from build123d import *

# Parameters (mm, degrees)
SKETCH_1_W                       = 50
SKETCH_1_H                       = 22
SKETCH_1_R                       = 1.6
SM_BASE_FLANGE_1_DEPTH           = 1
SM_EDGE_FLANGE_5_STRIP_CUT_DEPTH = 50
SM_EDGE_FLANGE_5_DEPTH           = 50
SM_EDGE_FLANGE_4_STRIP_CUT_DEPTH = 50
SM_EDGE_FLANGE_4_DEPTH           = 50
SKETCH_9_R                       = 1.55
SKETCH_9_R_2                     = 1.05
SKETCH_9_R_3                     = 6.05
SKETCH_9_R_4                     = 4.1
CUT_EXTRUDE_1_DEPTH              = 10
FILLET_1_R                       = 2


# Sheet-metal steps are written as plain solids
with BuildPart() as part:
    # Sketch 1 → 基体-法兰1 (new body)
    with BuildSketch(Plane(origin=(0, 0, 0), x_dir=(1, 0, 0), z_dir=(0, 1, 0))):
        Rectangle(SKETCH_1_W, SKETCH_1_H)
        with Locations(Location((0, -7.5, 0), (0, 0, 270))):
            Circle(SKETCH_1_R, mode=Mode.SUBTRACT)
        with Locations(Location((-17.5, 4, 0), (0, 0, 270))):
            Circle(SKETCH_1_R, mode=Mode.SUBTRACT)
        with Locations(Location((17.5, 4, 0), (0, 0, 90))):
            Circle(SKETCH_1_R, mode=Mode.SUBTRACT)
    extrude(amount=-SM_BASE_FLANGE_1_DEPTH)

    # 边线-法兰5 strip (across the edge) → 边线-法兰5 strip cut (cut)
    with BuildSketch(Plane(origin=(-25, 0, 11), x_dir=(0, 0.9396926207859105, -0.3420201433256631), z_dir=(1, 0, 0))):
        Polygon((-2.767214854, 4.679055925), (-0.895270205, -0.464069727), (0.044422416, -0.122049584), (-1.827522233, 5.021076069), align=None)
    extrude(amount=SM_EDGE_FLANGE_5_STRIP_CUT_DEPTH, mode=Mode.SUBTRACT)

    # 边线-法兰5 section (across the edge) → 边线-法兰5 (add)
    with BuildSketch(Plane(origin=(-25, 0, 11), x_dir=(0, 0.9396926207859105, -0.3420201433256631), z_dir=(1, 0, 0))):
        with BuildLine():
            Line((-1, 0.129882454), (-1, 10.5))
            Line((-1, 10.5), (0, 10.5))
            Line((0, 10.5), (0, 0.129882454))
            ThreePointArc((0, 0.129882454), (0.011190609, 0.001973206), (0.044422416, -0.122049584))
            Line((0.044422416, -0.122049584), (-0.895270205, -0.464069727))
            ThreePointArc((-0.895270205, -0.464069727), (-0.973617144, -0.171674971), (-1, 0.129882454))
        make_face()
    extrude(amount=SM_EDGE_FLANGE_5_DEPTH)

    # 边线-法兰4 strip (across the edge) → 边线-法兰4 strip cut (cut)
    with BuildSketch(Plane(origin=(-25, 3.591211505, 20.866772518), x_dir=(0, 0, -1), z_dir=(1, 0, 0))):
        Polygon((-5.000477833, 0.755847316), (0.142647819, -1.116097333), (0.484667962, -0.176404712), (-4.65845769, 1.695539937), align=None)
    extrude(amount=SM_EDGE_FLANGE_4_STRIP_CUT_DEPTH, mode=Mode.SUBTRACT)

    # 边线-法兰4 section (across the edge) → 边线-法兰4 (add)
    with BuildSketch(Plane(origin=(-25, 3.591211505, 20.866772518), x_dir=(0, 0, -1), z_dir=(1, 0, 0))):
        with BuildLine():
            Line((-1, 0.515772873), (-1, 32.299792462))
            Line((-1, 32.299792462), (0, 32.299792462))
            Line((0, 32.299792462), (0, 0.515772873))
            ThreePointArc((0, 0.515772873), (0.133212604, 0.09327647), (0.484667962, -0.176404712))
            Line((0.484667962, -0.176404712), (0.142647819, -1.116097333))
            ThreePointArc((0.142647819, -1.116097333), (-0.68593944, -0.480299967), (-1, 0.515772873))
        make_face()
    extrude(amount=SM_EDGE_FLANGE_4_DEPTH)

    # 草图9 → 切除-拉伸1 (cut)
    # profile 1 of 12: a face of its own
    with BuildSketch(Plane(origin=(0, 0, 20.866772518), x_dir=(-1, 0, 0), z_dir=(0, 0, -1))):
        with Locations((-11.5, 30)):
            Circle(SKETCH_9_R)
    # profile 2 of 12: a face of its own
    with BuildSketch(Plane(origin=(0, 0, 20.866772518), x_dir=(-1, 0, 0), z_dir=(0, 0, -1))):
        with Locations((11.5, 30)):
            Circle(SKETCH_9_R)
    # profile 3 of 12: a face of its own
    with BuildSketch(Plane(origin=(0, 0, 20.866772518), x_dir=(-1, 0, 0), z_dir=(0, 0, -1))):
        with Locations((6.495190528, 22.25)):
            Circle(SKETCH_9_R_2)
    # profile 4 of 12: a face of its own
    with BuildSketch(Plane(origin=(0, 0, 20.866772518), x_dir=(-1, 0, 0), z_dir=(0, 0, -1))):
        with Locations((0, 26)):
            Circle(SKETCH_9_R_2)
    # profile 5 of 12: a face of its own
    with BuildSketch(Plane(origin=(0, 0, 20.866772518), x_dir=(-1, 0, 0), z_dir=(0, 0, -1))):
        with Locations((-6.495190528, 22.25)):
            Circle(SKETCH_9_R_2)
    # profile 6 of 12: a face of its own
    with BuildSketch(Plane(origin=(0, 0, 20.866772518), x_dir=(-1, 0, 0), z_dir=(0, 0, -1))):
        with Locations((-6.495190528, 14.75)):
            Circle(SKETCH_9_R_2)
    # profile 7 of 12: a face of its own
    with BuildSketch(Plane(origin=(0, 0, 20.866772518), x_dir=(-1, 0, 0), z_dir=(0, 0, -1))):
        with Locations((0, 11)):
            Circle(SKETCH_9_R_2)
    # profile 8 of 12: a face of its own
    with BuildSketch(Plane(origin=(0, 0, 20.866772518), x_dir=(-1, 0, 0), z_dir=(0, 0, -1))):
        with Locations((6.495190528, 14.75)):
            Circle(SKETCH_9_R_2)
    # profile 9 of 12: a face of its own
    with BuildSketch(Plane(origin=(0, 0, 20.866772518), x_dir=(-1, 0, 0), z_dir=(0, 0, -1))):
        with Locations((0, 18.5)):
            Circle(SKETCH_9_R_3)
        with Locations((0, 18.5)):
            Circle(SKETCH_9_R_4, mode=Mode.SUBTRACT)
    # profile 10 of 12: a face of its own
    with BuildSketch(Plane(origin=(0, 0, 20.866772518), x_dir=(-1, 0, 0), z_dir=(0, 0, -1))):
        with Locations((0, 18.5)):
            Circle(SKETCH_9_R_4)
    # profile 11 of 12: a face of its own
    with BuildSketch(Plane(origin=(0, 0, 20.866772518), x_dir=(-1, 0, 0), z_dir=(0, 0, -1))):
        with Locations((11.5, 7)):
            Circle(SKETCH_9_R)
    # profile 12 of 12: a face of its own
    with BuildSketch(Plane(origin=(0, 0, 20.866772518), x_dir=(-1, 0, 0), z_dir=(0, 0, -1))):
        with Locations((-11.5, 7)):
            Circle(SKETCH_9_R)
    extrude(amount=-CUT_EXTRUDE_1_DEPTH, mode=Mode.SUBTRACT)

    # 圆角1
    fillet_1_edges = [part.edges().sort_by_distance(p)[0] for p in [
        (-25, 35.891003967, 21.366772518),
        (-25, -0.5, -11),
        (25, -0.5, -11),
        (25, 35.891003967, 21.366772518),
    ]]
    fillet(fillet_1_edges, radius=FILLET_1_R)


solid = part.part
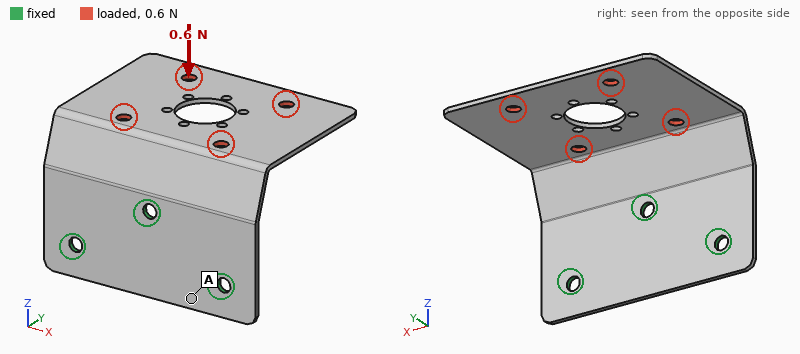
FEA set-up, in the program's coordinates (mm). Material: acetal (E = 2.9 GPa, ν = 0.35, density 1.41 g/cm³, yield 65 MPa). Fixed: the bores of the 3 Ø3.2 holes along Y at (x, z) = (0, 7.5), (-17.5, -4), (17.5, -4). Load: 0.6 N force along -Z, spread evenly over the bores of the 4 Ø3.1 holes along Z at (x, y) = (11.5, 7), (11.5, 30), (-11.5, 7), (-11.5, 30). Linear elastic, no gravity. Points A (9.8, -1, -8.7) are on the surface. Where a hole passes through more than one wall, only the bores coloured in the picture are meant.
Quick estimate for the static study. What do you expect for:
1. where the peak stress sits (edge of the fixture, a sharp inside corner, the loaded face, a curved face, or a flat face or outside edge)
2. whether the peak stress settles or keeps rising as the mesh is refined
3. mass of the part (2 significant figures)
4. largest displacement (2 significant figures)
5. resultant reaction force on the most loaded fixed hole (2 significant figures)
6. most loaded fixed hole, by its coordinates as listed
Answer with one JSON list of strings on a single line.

["edge of the fixture", "keeps rising", "4.3 g", "0.69 mm", "1.1 N", "(0, 7.5)"]
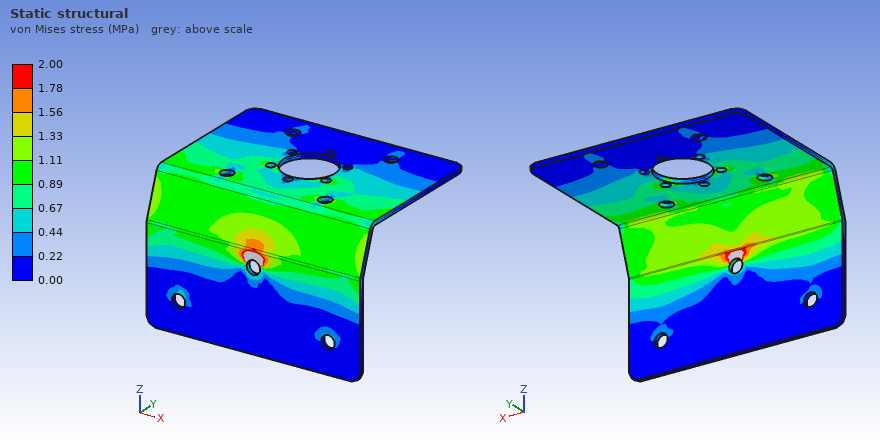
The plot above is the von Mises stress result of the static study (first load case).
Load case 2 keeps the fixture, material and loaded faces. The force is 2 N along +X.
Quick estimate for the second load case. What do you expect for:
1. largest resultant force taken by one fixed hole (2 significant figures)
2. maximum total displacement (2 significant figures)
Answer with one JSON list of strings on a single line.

["1.2 N", "0.72 mm"]
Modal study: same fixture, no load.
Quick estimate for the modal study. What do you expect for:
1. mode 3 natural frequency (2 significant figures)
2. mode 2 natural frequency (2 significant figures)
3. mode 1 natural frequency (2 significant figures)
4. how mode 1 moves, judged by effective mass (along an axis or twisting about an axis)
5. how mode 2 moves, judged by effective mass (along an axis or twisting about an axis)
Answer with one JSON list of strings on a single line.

["340 Hz", "180 Hz", "120 Hz", "along Z", "along X"]
